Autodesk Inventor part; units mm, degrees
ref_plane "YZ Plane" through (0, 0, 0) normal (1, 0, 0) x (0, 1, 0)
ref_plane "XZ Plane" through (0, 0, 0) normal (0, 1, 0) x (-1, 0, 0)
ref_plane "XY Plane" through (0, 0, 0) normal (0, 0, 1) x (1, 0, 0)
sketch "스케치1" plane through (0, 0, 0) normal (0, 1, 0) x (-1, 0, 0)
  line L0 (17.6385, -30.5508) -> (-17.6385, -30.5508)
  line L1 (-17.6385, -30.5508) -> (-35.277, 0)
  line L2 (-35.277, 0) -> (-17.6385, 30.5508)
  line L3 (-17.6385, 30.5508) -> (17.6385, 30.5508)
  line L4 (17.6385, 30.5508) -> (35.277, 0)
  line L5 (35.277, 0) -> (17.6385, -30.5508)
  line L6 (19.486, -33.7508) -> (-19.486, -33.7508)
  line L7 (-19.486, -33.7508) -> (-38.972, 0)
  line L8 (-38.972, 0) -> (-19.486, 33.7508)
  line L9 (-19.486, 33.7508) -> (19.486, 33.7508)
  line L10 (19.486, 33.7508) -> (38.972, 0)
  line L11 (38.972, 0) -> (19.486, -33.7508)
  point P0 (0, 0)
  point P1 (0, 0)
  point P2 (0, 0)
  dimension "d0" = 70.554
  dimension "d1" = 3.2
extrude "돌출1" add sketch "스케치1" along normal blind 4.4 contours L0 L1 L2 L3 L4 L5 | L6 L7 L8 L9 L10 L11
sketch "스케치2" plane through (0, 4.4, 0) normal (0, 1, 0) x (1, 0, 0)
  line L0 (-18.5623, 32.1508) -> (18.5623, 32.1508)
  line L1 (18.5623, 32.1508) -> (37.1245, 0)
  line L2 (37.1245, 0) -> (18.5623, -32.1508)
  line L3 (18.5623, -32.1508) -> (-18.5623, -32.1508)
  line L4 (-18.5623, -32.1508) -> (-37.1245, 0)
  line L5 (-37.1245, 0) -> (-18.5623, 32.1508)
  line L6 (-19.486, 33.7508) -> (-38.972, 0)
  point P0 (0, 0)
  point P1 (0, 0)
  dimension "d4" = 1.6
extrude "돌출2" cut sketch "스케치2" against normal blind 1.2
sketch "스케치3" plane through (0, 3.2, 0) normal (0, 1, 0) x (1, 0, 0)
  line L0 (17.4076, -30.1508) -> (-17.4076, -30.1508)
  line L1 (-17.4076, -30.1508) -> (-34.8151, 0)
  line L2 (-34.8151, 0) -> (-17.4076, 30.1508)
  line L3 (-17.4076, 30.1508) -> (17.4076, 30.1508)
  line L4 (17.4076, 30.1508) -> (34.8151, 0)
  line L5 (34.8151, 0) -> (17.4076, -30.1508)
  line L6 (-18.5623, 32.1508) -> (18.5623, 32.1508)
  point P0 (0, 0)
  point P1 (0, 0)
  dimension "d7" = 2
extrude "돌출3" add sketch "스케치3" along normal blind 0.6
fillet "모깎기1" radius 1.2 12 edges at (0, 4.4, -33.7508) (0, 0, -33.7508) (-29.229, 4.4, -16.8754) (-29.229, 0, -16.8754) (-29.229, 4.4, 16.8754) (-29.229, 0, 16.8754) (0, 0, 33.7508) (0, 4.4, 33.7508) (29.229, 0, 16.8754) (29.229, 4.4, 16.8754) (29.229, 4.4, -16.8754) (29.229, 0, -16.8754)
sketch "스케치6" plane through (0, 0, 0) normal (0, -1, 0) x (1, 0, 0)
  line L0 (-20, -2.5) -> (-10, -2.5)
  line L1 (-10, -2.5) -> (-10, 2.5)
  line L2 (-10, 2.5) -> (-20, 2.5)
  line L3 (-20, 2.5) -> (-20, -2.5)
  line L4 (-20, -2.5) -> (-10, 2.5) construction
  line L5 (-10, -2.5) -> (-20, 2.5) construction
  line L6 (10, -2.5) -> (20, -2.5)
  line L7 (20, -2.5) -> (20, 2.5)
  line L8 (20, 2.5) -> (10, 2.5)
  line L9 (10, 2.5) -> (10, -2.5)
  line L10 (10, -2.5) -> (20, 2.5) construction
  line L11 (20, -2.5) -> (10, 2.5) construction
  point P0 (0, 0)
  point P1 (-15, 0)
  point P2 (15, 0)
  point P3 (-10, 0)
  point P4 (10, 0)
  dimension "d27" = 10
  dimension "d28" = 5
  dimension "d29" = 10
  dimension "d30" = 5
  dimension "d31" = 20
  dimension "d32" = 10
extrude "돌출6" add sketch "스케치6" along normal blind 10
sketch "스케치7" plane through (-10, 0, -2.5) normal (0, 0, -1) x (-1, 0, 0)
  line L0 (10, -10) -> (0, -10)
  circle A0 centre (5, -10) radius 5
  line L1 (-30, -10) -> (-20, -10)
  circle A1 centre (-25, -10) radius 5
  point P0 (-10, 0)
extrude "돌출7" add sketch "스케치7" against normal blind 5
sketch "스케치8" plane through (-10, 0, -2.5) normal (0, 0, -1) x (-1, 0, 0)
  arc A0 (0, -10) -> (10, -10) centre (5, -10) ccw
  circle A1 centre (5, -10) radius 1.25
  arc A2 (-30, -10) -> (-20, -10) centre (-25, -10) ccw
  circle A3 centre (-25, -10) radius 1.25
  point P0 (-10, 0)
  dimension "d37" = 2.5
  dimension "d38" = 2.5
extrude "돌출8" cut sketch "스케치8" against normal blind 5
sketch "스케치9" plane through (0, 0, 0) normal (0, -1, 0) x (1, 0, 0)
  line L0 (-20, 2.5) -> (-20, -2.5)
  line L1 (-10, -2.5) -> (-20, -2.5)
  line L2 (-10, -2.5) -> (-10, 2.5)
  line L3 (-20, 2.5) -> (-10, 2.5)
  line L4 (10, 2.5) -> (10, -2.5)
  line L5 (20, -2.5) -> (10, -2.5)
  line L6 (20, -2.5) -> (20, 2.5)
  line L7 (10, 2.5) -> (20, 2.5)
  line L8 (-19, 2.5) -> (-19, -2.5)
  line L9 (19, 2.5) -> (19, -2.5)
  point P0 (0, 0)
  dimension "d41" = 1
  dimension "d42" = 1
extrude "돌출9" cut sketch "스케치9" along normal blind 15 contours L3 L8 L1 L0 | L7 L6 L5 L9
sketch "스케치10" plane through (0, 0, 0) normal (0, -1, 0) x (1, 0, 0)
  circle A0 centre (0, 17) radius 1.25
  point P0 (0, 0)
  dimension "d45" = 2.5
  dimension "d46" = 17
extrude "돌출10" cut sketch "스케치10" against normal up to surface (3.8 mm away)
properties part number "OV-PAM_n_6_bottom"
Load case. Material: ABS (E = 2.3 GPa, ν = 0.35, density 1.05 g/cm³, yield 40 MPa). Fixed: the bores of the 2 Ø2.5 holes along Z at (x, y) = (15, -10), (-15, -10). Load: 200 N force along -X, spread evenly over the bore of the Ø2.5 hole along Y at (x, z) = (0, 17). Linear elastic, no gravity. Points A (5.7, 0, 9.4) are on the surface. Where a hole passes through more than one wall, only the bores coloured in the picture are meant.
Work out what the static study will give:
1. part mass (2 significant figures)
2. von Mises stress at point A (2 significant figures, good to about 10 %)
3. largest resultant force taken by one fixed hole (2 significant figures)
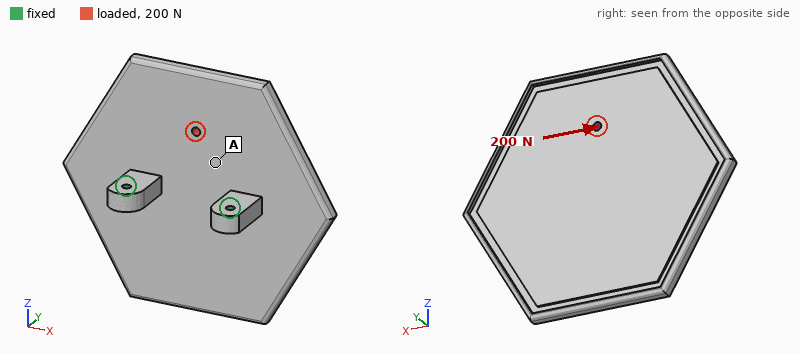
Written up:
17 g
4.4 MPa
150 N
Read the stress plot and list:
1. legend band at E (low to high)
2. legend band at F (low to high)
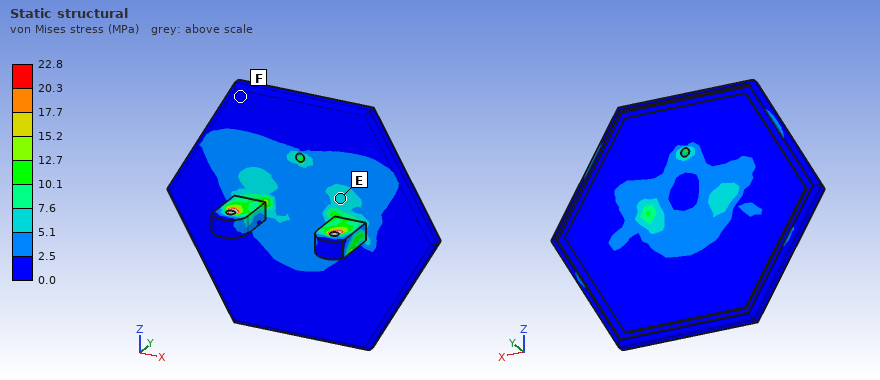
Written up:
5.1 to 7.6 MPa
0.0 to 2.5 MPa
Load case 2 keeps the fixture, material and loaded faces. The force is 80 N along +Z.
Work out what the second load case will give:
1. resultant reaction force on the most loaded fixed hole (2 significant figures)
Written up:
40 N
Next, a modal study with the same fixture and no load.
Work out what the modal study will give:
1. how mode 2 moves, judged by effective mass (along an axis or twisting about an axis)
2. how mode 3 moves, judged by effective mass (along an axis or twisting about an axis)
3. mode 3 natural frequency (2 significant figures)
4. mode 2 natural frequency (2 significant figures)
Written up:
twisting about Y
along Y
970 Hz
870 Hz
